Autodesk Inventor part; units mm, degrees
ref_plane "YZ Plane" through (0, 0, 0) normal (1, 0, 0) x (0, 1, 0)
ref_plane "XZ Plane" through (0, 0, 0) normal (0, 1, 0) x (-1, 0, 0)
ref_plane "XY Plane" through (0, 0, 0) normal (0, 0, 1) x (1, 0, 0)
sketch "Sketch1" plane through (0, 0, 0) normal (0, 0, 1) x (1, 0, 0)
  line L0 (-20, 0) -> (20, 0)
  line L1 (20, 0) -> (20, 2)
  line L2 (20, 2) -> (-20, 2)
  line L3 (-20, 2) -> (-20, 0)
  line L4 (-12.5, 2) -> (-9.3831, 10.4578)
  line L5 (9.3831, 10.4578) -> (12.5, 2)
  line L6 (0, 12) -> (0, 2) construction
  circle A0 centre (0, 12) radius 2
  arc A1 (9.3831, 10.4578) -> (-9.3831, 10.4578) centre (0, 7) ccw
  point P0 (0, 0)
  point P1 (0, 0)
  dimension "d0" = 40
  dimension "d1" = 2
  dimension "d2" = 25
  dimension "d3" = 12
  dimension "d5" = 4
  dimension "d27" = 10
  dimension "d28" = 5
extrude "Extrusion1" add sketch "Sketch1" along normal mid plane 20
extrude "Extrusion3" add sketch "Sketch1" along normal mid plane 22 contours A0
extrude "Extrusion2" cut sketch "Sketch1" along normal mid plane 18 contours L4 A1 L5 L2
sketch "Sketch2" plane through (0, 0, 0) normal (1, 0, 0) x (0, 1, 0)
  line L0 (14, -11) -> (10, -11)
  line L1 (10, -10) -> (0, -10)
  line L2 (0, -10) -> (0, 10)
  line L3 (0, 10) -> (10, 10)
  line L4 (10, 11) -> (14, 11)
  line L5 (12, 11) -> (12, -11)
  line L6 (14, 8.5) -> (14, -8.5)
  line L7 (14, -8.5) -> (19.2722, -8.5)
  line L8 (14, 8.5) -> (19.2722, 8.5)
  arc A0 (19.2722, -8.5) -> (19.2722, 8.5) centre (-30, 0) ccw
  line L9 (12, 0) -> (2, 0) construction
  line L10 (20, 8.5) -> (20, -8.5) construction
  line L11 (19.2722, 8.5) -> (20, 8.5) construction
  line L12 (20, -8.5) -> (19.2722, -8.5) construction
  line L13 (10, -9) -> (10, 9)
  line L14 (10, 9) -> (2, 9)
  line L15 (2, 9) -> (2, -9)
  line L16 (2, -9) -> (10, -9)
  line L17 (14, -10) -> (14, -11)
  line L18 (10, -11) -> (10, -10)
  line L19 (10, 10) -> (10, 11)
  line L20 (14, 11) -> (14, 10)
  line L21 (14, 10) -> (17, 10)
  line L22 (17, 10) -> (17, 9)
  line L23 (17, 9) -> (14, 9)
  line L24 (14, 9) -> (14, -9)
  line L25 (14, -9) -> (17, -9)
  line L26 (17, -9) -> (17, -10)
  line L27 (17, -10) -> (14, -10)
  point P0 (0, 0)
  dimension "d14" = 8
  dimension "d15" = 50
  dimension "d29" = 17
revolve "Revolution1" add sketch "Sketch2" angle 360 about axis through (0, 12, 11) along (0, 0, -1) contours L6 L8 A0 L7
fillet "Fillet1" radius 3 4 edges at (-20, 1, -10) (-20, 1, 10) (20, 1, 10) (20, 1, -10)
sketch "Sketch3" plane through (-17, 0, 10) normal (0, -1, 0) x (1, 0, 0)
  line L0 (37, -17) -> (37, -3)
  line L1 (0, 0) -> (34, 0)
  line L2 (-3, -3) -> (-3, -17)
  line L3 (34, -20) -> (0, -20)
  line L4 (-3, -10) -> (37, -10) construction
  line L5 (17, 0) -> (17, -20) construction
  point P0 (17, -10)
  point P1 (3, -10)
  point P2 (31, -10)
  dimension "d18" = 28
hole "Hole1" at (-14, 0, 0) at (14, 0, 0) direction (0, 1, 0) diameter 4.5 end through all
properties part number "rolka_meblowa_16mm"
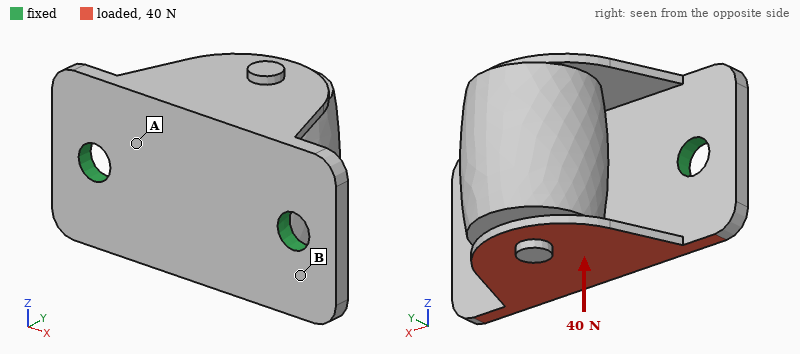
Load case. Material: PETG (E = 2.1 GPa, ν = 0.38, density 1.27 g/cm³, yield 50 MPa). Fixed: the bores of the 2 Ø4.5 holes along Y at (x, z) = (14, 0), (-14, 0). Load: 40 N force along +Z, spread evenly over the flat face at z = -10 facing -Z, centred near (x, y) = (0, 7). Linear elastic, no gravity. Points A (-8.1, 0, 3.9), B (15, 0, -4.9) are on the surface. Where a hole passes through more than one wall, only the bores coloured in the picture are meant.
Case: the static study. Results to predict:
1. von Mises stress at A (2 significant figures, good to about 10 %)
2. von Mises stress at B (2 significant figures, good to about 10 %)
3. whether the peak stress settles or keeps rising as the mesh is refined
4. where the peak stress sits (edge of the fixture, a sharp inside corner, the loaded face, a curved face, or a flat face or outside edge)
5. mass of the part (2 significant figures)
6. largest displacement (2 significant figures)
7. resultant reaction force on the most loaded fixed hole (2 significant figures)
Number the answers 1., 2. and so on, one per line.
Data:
1. 2.4 MPa
2. 4.5 MPa
3. keeps rising
4. a sharp inside corner
5. 6.8 g
6. 0.52 mm
7. 20 N
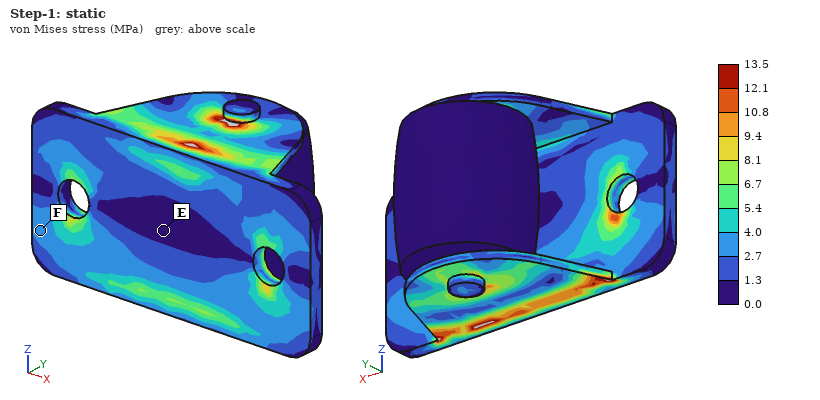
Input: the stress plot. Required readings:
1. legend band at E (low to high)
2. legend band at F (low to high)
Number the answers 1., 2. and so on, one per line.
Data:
1. 0.0 to 1.3 MPa
2. 2.7 to 4.0 MPa
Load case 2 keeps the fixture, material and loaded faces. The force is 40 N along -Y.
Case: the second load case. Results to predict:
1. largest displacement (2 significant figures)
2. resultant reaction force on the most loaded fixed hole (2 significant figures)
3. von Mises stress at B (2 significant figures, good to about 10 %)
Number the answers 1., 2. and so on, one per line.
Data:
1. 0.36 mm
2. 20 N
3. 10 MPa
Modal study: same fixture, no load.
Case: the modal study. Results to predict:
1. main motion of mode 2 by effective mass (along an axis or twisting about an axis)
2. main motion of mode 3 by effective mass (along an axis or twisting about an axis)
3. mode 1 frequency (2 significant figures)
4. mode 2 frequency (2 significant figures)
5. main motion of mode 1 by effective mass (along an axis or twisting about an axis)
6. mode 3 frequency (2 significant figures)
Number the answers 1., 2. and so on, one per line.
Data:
1. along X
2. along Y
3. 520 Hz
4. 1300 Hz
5. along Z
6. 1400 Hz
